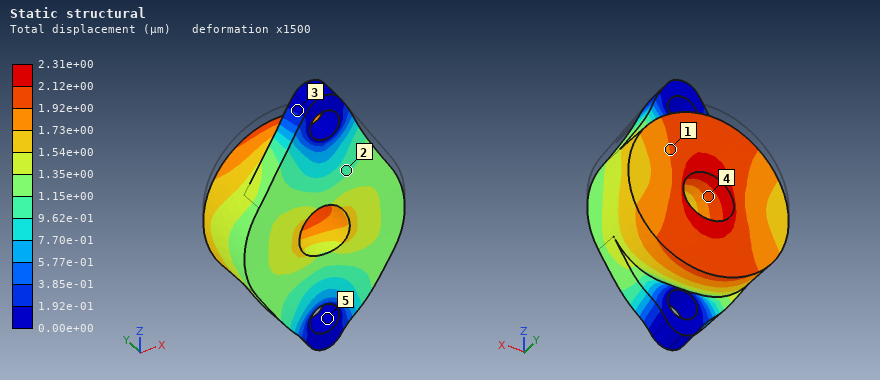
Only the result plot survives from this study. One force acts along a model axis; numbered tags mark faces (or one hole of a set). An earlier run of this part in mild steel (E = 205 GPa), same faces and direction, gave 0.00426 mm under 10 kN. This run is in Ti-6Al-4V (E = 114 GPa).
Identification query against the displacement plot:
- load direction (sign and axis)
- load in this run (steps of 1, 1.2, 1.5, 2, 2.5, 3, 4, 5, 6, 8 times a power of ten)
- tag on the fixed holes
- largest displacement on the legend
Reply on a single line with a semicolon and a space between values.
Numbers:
-Z; 3 kN; 5; 2.31e+00 µm
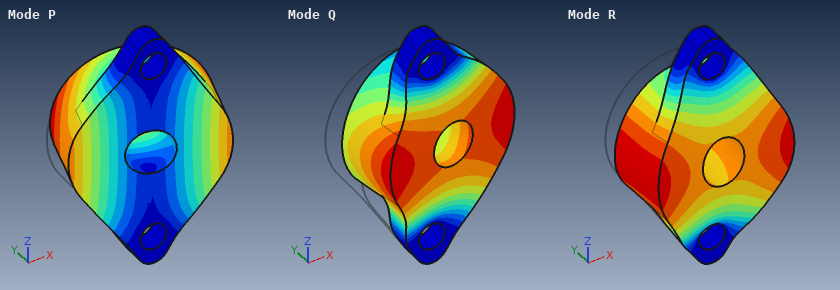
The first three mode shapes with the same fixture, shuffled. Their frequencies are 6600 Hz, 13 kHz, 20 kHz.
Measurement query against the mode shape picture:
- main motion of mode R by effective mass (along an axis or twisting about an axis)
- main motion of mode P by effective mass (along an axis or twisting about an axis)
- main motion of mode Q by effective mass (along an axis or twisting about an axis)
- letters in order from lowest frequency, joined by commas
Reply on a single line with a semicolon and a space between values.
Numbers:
along Y; along X; along X; P, R, Q
